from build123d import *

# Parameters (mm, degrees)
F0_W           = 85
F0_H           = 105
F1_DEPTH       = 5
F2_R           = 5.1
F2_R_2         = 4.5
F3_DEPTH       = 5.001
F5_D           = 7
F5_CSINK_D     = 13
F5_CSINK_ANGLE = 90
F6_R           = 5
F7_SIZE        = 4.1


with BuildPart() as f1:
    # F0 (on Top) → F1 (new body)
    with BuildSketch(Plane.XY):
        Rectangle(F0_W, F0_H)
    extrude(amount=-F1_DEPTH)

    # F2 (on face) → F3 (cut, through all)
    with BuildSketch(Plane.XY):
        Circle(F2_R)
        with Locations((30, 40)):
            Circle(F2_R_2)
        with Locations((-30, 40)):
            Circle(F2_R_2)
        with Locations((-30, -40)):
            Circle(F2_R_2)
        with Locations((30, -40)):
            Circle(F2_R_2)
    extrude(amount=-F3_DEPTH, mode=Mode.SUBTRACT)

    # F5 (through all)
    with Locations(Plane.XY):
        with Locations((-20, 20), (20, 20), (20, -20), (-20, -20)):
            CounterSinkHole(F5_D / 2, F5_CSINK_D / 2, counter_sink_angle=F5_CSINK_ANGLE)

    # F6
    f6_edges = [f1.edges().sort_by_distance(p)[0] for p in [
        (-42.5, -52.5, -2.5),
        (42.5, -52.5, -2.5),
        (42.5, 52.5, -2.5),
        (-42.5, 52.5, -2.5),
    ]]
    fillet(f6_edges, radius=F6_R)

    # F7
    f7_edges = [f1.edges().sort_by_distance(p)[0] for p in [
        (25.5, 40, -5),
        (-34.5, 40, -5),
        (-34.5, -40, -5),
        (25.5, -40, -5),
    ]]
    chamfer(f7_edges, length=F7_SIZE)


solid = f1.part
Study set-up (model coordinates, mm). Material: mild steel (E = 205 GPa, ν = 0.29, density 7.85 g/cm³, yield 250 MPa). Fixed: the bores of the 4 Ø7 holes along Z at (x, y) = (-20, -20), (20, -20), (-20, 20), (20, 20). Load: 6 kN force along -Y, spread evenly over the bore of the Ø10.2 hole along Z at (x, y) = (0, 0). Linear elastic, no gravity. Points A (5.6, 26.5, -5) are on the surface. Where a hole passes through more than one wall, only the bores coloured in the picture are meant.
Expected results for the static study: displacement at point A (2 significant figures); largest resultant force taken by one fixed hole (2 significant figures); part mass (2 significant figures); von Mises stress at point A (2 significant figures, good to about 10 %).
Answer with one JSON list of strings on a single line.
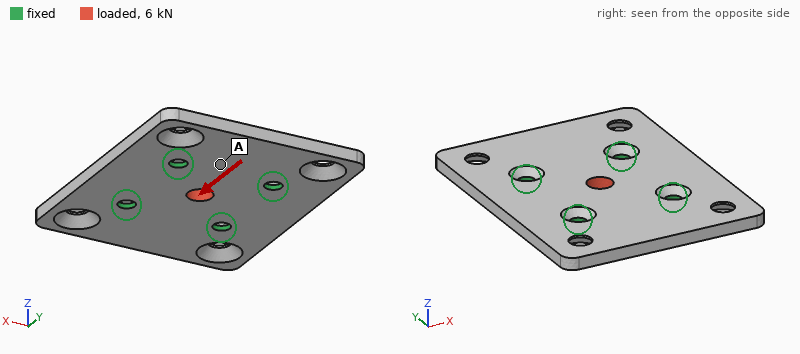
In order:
["1.3 µm", "1.5 kN", "320 g", "9.6 MPa"]
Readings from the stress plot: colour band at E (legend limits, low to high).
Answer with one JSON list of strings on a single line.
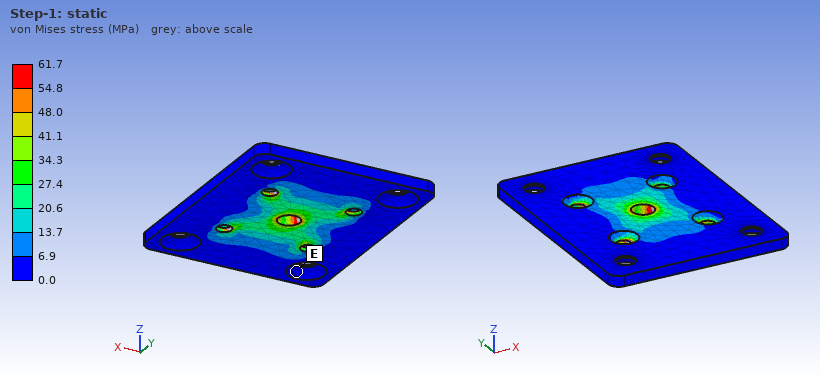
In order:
["0.0 to 6.9 MPa"]
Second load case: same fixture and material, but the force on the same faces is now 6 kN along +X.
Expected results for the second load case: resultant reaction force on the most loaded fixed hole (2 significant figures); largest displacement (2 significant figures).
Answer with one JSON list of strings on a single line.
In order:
["1.6 kN", "3.6 µm"]
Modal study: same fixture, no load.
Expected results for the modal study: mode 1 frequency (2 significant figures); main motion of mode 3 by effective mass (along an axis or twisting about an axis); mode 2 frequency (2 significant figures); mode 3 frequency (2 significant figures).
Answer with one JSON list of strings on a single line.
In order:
["3100 Hz", "twisting about Y", "3200 Hz", "4100 Hz"]
